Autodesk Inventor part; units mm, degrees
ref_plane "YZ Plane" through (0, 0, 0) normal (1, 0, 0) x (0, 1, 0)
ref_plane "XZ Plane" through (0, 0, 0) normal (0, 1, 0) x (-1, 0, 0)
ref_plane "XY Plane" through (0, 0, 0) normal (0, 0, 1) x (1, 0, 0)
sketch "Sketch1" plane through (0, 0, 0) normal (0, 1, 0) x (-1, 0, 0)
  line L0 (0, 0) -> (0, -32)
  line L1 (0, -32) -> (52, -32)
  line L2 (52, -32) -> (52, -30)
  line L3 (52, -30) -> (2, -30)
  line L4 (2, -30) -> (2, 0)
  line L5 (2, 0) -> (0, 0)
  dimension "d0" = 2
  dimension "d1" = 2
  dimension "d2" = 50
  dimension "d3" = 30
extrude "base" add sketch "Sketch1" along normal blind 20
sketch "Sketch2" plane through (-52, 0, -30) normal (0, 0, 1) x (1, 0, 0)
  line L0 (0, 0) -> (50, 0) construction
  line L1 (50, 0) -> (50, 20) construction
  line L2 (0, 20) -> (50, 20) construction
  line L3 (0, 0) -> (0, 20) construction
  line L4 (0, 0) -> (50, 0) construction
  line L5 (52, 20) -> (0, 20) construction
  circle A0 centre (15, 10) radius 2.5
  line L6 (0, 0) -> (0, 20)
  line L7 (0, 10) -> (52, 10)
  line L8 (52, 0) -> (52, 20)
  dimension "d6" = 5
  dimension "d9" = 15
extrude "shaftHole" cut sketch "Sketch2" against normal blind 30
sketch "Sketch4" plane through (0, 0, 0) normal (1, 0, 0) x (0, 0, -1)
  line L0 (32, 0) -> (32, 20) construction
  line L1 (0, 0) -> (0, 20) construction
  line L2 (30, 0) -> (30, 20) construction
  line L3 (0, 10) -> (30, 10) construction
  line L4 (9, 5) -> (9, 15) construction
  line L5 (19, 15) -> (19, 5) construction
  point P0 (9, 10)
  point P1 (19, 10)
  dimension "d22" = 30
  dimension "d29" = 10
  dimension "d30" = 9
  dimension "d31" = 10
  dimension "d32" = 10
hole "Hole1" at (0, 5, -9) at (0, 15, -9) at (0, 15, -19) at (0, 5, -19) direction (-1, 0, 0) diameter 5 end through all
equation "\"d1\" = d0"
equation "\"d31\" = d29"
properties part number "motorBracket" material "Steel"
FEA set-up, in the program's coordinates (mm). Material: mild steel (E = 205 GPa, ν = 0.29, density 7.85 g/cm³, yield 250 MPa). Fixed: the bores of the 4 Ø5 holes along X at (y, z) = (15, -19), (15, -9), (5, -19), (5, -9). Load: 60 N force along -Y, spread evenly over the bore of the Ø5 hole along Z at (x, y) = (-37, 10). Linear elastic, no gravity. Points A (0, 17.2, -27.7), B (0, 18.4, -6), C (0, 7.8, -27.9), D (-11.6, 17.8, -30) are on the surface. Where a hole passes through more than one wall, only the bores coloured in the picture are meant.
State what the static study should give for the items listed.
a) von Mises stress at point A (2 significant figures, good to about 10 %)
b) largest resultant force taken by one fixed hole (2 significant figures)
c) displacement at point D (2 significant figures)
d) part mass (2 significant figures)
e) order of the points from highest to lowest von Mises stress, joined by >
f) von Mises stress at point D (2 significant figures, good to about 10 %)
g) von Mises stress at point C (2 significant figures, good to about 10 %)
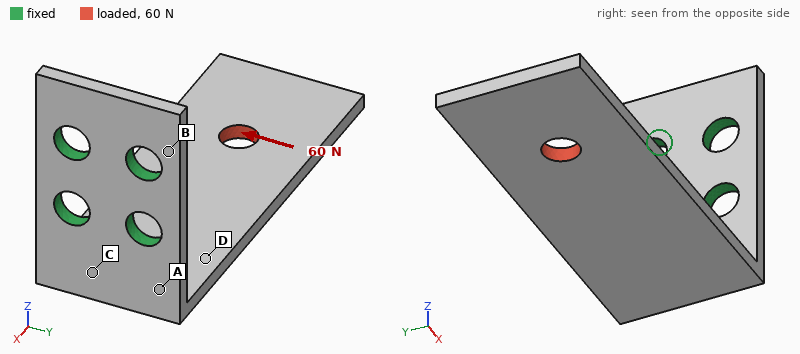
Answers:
63 MPa
170 N
0.033 mm
24 g
C > A > D > B
19 MPa
75 MPa
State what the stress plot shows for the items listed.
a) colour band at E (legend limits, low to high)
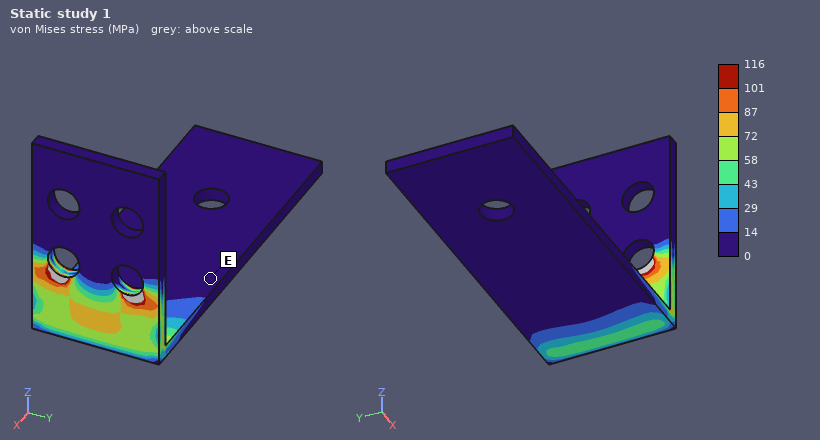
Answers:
0 to 14 MPa
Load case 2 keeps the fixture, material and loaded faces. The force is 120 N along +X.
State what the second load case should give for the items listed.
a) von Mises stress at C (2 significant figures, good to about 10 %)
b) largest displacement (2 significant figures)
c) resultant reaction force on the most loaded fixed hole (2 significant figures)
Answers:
25 MPa
0.11 mm
61 N
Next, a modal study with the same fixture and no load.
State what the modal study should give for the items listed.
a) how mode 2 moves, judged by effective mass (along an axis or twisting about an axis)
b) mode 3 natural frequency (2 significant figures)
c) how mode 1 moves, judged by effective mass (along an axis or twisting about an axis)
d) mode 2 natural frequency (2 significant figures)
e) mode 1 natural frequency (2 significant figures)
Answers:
along Y
3000 Hz
along Z
1300 Hz
500 Hz
